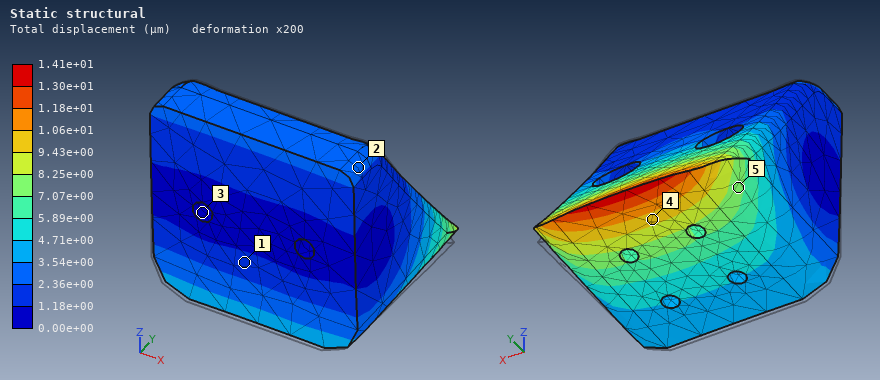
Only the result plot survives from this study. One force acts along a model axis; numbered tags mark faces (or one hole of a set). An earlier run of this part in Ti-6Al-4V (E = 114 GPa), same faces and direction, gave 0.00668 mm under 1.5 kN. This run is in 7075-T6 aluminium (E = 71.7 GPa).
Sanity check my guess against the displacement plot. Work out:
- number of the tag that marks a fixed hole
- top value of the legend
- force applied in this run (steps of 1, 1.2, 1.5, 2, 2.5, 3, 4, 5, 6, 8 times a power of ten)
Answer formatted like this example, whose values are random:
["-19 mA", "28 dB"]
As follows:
["3", "1.41e+01 µm", "2 kN"]
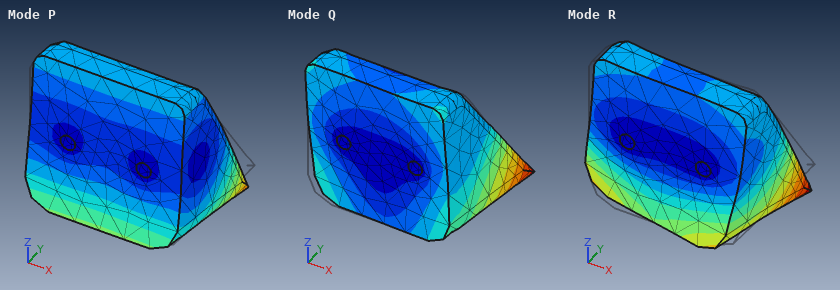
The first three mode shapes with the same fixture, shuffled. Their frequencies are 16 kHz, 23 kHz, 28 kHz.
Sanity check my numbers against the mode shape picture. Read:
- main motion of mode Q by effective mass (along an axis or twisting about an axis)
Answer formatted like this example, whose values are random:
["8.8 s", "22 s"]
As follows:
["along X"]
